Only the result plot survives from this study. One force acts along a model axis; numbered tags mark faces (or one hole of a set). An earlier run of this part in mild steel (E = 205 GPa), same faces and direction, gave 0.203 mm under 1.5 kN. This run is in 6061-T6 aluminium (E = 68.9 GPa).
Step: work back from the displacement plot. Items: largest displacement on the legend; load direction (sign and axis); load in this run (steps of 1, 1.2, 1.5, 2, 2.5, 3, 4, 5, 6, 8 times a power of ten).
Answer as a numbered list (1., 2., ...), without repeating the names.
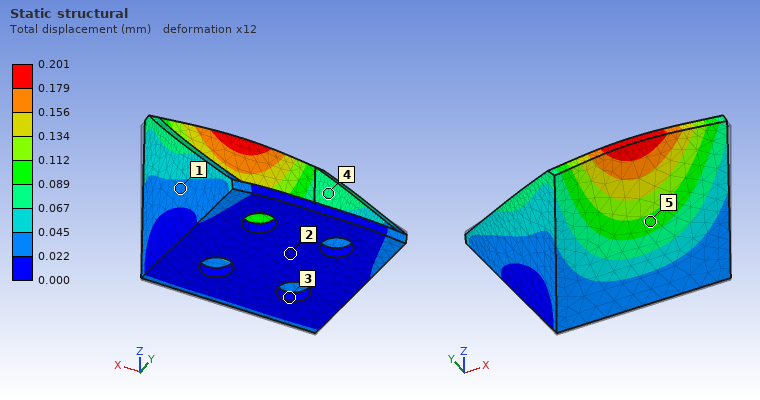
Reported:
1. 0.201 mm
2. +Y
3. 500 N
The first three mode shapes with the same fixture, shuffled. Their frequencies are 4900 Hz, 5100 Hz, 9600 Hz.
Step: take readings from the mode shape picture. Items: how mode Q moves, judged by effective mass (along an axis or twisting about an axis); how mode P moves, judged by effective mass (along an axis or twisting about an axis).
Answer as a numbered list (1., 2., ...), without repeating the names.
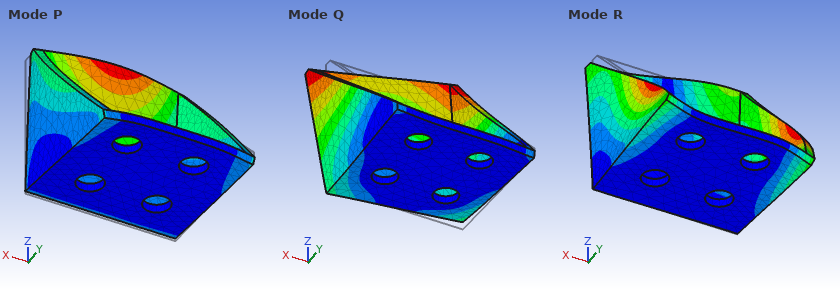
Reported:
1. along X
2. along Y
